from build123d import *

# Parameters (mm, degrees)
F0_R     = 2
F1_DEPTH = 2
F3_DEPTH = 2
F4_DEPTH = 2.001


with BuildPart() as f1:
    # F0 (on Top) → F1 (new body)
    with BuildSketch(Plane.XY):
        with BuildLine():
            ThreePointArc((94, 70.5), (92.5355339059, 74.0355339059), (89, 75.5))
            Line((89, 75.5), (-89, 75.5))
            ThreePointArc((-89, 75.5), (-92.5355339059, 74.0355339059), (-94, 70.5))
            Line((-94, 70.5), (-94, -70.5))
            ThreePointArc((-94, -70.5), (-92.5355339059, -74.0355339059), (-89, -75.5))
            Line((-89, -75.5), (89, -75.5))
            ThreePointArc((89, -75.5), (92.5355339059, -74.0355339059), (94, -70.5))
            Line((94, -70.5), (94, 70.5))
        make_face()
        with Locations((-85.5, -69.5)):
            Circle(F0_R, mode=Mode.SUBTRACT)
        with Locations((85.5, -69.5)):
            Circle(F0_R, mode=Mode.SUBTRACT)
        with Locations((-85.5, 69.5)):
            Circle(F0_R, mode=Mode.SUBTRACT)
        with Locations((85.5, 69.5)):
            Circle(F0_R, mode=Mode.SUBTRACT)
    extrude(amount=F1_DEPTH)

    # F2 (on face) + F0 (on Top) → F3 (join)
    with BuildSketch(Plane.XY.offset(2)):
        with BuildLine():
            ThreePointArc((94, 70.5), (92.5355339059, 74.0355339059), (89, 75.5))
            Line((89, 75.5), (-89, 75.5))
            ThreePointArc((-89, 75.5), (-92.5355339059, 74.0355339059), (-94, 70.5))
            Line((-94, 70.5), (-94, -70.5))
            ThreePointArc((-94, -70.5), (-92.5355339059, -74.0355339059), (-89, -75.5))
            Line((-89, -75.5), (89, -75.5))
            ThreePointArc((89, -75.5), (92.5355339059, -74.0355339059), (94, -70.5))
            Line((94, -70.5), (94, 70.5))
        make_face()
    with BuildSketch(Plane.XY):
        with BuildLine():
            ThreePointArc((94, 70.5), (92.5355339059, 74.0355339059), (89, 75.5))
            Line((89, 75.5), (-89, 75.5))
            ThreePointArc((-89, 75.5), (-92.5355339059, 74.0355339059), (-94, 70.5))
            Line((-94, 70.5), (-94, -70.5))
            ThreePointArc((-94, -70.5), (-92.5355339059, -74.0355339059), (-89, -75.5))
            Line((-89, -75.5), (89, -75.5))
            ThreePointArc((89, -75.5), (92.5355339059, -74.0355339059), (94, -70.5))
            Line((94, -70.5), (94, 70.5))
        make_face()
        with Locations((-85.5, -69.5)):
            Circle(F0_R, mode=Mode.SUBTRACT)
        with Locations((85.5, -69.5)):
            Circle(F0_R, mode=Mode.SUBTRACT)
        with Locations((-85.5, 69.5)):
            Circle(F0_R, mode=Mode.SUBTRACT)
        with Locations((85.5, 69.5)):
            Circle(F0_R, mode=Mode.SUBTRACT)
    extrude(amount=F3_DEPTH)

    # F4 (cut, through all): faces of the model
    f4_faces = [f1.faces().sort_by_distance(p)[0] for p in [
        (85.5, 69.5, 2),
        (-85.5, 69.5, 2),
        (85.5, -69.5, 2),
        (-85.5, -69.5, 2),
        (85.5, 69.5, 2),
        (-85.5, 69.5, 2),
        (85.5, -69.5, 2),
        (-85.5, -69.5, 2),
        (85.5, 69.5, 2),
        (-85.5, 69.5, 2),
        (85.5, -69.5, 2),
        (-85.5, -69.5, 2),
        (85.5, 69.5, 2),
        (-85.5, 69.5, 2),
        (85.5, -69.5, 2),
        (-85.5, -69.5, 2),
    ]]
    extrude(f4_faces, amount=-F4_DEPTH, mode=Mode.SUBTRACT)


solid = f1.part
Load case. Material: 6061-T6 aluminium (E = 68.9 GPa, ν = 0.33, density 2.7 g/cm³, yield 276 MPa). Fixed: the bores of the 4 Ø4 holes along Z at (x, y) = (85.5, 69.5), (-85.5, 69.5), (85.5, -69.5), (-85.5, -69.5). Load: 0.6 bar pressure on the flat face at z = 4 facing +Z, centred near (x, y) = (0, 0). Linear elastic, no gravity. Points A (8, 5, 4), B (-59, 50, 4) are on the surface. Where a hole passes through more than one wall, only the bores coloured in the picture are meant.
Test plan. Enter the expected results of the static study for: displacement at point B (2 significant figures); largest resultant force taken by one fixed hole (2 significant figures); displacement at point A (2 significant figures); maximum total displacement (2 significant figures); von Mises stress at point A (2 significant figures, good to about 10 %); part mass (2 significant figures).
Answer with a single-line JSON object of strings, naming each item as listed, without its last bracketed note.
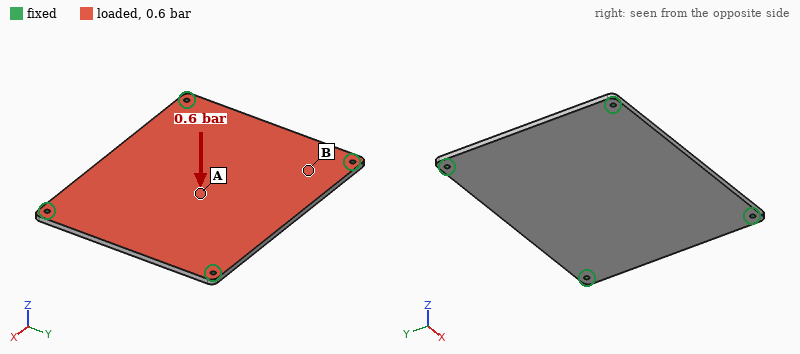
{"displacement at point B": "0.33 mm", "largest resultant force taken by one fixed hole": "420 N", "displacement at point A": "0.84 mm", "maximum total displacement": "0.84 mm", "von Mises stress at point A": "35 MPa", "part mass": "310 g"}
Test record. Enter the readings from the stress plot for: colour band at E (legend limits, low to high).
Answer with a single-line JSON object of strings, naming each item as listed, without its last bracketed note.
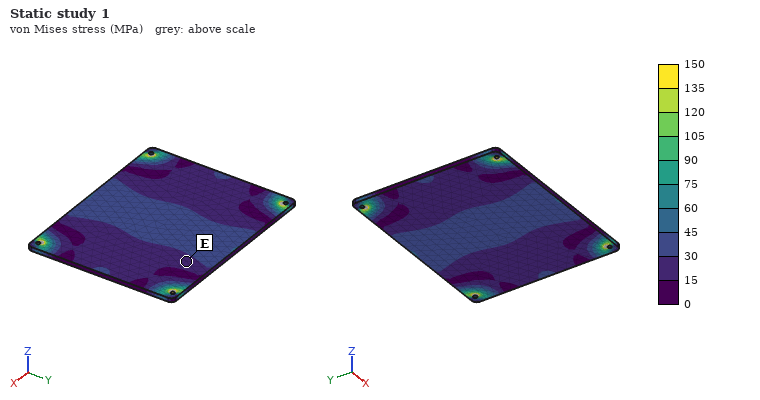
{"colour band at E": "15 to 30 MPa"}
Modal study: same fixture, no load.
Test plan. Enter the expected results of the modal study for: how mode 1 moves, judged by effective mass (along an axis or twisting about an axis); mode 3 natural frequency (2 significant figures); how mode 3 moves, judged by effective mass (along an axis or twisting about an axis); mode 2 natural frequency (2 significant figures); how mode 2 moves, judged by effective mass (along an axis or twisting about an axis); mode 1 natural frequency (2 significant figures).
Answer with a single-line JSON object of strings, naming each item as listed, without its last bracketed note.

{"how mode 1 moves, judged by effective mass": "along Z", "mode 3 natural frequency": "1000 Hz", "how mode 3 moves, judged by effective mass": "twisting about Y", "mode 2 natural frequency": "830 Hz", "how mode 2 moves, judged by effective mass": "twisting about X", "mode 1 natural frequency": "480 Hz"}
